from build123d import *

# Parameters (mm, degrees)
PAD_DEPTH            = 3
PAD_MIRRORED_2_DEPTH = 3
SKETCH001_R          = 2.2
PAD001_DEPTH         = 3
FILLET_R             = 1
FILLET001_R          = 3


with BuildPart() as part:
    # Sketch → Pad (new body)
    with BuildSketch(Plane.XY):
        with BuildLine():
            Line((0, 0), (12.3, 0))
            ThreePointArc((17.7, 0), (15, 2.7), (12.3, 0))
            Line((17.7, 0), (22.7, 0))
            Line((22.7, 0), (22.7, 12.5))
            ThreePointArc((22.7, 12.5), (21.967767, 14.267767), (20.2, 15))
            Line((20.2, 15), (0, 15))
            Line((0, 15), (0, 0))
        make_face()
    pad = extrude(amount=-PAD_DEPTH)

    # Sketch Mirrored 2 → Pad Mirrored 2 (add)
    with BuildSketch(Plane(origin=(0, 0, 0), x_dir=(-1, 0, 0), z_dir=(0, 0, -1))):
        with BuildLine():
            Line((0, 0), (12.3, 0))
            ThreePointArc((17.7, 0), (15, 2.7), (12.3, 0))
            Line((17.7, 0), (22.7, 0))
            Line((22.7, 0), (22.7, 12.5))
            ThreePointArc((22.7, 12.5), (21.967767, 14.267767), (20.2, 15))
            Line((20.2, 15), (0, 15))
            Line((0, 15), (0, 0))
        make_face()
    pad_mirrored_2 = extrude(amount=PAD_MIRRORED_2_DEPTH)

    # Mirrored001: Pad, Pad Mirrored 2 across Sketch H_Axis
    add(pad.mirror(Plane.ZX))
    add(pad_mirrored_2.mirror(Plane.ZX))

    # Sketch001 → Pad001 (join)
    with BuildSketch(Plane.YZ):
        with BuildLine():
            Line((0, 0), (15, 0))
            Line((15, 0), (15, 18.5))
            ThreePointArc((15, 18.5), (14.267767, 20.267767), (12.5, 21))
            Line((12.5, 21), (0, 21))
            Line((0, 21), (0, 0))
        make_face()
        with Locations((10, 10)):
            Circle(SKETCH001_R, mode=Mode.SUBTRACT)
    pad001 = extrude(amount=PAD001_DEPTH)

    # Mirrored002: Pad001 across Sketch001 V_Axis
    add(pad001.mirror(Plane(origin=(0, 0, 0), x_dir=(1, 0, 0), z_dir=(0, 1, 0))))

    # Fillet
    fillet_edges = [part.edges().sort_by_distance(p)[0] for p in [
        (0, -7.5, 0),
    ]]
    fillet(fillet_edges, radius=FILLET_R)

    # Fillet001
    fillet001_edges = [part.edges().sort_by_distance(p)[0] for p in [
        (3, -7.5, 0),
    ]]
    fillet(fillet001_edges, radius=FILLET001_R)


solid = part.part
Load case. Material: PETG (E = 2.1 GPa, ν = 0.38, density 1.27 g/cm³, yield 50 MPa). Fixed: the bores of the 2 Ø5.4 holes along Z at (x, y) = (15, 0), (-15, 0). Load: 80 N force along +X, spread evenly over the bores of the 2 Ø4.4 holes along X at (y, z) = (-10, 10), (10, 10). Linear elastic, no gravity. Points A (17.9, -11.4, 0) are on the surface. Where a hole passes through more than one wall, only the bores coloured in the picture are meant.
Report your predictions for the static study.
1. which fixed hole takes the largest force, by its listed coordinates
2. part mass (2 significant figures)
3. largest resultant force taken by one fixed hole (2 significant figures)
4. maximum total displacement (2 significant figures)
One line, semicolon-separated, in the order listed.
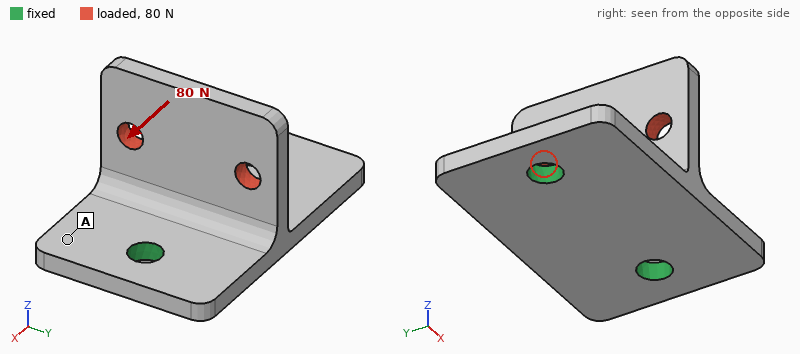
(15, 0); 7.4 g; 63 N; 0.64 mm
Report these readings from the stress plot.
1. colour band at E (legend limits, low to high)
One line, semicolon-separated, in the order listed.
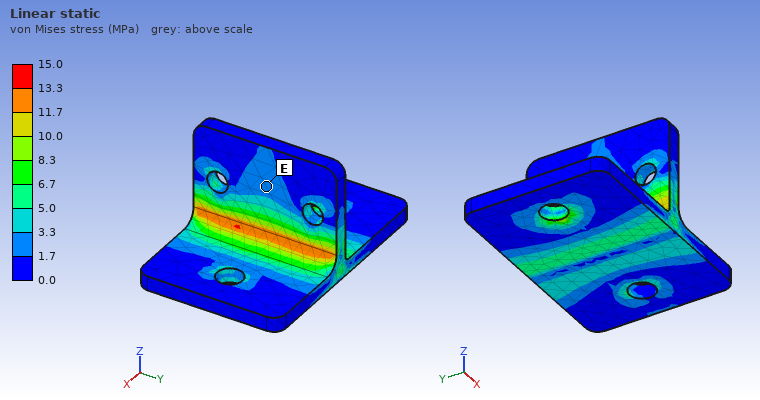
1.7 to 3.3 MPa
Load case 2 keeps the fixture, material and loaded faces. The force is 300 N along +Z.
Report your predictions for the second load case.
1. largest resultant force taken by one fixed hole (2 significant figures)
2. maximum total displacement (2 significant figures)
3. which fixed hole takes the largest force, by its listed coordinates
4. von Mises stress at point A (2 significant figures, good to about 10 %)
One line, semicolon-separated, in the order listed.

170 N; 0.37 mm; (15, 0); 3.4 MPa
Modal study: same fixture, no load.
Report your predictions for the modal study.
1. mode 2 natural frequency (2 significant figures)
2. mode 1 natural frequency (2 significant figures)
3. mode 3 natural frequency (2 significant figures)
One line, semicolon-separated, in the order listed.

1300 Hz; 1300 Hz; 2400 Hz
